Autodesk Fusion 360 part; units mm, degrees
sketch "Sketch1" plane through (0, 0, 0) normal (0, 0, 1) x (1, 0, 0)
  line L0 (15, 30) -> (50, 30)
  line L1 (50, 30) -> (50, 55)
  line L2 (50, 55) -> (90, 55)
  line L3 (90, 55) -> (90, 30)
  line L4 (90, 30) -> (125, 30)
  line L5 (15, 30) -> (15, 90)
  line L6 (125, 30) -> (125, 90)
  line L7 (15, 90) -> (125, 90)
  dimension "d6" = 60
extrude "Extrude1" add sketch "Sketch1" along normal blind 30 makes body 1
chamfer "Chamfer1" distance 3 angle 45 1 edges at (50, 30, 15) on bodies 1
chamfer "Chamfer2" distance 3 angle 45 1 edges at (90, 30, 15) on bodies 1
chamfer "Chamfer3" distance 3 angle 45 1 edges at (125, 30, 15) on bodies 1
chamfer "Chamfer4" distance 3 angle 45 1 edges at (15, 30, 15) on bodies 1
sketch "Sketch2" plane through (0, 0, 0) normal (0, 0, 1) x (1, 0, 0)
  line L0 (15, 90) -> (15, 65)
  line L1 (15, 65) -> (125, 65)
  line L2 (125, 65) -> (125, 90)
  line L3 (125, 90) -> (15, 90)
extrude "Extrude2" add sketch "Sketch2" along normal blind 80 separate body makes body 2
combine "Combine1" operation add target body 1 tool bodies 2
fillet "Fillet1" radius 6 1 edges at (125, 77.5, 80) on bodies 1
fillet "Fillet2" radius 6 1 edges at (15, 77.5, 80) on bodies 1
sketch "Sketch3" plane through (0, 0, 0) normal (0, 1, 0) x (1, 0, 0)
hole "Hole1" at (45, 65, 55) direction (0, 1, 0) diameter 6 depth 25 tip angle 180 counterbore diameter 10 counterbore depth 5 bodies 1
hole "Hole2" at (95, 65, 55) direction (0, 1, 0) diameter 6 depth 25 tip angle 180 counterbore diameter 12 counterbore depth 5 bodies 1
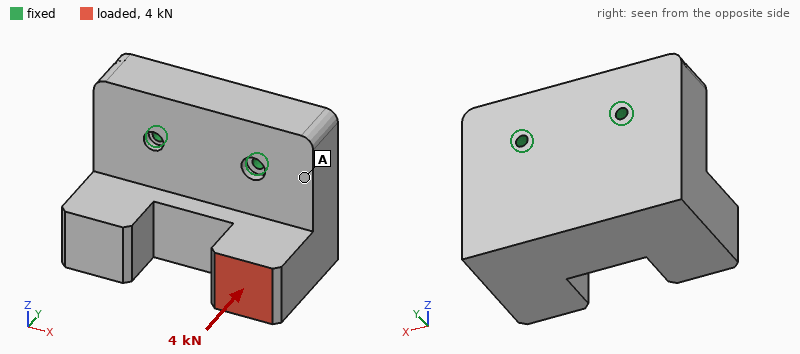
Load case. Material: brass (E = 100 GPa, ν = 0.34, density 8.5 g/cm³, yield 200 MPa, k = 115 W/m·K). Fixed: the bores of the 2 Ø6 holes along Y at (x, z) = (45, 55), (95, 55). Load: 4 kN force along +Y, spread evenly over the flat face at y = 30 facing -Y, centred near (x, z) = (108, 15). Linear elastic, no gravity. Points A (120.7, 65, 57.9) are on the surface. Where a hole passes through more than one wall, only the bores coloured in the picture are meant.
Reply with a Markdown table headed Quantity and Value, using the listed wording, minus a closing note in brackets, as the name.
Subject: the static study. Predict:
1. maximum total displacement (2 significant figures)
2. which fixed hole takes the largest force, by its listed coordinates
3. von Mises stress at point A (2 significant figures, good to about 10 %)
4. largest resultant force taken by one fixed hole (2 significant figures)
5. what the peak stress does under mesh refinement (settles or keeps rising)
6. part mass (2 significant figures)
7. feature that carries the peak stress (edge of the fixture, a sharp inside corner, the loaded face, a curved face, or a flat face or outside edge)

| Quantity | Value |
|---|---|
| maximum total displacement | 52 µm |
| which fixed hole takes the largest force, by its listed coordinates | (95, 55) |
| von Mises stress at point A | 7.8 MPa |
| largest resultant force taken by one fixed hole | 4.3 kN |
| what the peak stress does under mesh refinement | keeps rising |
| part mass | 2.6 kg |
| feature that carries the peak stress | edge of the fixture |
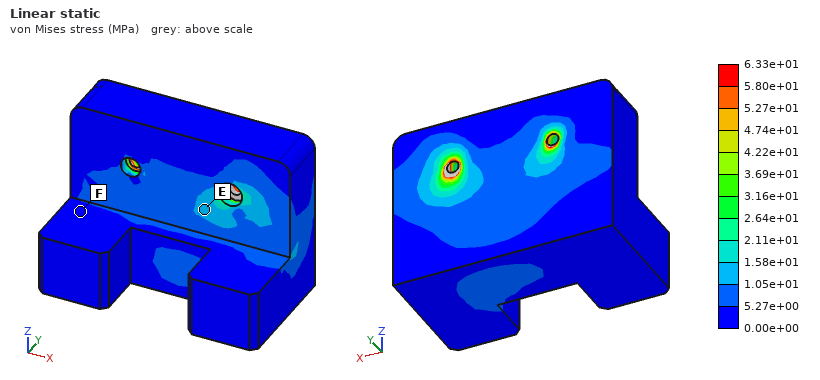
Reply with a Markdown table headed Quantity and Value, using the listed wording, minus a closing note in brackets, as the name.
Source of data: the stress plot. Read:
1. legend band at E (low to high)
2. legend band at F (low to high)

| Quantity | Value |
|---|---|
| legend band at E | 1.05e+01 to 1.58e+01 MPa |
| legend band at F | 0.00e+00 to 5.27e+00 MPa |
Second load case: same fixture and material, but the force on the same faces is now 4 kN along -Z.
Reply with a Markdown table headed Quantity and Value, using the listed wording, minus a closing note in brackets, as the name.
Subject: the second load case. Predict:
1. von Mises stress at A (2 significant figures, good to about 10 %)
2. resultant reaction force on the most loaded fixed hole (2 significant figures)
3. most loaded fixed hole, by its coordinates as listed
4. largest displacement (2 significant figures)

| Quantity | Value |
|---|---|
| von Mises stress at A | 10 MPa |
| resultant reaction force on the most loaded fixed hole | 4.9 kN |
| most loaded fixed hole, by its coordinates as listed | (95, 55) |
| largest displacement | 85 µm |
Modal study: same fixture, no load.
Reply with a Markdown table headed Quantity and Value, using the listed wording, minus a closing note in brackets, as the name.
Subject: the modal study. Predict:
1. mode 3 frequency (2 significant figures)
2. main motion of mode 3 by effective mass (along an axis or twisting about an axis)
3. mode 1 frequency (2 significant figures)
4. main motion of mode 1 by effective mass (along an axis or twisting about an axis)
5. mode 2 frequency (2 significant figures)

| Quantity | Value |
|---|---|
| mode 3 frequency | 3500 Hz |
| main motion of mode 3 by effective mass | along X |
| mode 1 frequency | 1600 Hz |
| main motion of mode 1 by effective mass | along Y |
| mode 2 frequency | 2600 Hz |
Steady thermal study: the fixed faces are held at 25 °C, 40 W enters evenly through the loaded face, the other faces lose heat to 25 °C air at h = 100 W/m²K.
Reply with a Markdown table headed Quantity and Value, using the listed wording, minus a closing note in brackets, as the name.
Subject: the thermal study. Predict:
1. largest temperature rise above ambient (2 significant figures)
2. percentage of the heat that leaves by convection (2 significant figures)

| Quantity | Value |
|---|---|
| largest temperature rise above ambient | 19 K |
| percentage of the heat that leaves by convection | 33 % |
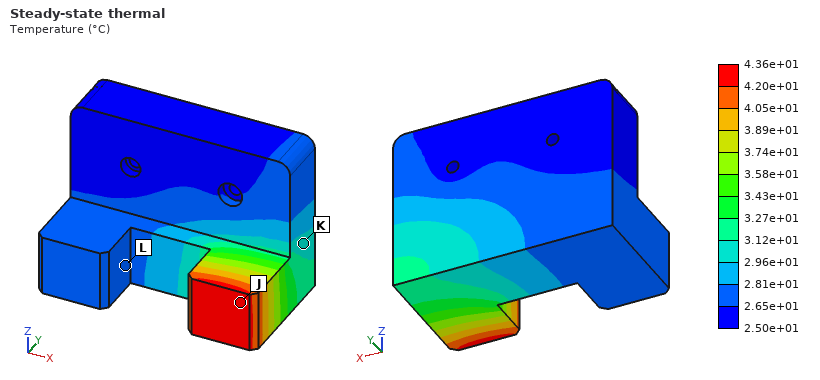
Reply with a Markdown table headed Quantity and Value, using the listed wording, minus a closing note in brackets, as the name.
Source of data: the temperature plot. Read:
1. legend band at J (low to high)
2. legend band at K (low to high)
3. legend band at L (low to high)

| Quantity | Value |
|---|---|
| legend band at J | 4.20e+01 to 4.36e+01 °C |
| legend band at K | 2.96e+01 to 3.12e+01 °C |
| legend band at L | 2.65e+01 to 2.81e+01 °C |
